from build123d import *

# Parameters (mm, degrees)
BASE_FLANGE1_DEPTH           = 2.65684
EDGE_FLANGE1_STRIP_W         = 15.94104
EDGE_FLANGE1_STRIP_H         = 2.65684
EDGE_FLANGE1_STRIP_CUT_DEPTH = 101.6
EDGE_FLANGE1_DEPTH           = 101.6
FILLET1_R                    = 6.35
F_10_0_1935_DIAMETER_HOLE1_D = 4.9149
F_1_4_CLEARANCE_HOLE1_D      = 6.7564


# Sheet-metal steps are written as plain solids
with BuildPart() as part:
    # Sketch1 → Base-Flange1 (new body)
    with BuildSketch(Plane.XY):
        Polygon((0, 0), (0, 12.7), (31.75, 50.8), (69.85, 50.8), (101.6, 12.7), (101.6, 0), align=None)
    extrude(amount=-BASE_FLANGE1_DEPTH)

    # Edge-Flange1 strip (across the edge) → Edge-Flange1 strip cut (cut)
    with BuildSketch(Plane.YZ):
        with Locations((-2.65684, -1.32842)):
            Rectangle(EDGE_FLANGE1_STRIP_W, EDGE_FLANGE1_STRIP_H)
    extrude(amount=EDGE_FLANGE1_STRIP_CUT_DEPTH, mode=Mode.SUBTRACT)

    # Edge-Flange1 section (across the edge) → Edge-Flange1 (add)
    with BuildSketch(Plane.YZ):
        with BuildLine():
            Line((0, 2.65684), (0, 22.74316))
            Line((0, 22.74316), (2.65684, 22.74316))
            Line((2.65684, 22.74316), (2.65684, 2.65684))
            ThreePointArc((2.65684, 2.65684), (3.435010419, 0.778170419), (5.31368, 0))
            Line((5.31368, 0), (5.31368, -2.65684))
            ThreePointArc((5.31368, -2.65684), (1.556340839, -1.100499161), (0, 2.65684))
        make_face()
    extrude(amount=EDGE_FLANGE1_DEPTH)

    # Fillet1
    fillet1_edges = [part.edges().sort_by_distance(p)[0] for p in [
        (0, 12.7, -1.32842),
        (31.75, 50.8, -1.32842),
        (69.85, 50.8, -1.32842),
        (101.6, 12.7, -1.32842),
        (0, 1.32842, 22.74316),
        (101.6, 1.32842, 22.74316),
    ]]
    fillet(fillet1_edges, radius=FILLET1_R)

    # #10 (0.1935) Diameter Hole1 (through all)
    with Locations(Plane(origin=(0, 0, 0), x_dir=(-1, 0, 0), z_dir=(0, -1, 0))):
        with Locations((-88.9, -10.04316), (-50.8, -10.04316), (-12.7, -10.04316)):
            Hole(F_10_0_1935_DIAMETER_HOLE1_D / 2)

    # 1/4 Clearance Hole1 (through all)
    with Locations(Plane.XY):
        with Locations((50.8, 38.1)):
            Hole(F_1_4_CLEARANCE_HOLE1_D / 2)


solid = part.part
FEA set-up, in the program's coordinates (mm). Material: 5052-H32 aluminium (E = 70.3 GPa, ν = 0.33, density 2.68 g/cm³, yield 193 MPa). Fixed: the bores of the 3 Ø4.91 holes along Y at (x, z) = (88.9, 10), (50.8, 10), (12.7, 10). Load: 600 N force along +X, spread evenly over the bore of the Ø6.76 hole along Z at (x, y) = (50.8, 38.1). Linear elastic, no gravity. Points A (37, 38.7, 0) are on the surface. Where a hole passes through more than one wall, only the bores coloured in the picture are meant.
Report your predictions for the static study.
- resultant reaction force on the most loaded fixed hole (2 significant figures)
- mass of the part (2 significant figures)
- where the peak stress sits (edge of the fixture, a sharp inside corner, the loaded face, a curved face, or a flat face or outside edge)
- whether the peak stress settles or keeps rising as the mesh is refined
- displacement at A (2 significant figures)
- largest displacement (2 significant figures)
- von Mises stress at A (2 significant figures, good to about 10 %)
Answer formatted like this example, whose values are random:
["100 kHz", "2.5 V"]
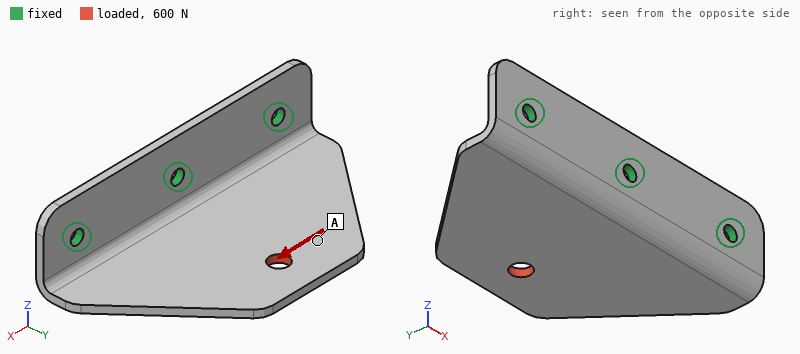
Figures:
["350 N", "43 g", "edge of the fixture", "keeps rising", "52 µm", "82 µm", "8.2 MPa"]
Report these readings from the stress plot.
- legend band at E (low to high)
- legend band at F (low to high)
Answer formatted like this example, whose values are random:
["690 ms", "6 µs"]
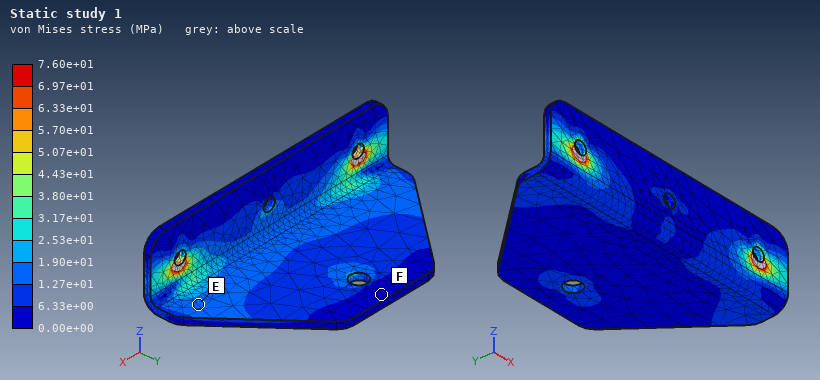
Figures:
["1.27e+01 to 1.90e+01 MPa", "0.00e+00 to 6.33e+00 MPa"]
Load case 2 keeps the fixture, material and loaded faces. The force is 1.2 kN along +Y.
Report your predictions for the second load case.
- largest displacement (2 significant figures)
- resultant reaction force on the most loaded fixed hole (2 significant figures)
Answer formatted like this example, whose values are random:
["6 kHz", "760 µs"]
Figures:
["0.37 mm", "450 N"]
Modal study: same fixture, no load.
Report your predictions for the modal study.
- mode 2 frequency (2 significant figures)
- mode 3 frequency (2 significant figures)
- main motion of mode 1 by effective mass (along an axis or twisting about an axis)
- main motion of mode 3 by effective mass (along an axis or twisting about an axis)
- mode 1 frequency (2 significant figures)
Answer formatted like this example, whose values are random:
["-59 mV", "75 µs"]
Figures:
["2100 Hz", "3800 Hz", "along Z", "along Y", "890 Hz"]
